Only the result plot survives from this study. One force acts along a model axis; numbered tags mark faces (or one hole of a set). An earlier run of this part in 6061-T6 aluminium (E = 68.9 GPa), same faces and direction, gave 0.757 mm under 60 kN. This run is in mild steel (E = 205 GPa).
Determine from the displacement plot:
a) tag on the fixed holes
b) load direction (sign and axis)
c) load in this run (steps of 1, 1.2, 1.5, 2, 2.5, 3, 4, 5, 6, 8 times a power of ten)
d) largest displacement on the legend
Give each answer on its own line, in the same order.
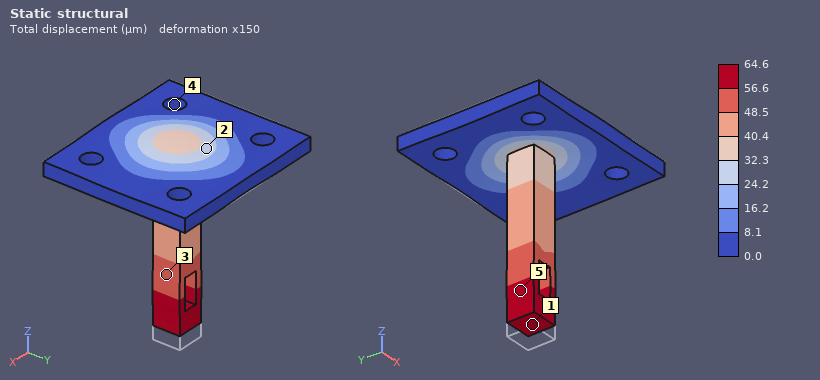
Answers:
4
+Z
15 kN
64.6 µm
